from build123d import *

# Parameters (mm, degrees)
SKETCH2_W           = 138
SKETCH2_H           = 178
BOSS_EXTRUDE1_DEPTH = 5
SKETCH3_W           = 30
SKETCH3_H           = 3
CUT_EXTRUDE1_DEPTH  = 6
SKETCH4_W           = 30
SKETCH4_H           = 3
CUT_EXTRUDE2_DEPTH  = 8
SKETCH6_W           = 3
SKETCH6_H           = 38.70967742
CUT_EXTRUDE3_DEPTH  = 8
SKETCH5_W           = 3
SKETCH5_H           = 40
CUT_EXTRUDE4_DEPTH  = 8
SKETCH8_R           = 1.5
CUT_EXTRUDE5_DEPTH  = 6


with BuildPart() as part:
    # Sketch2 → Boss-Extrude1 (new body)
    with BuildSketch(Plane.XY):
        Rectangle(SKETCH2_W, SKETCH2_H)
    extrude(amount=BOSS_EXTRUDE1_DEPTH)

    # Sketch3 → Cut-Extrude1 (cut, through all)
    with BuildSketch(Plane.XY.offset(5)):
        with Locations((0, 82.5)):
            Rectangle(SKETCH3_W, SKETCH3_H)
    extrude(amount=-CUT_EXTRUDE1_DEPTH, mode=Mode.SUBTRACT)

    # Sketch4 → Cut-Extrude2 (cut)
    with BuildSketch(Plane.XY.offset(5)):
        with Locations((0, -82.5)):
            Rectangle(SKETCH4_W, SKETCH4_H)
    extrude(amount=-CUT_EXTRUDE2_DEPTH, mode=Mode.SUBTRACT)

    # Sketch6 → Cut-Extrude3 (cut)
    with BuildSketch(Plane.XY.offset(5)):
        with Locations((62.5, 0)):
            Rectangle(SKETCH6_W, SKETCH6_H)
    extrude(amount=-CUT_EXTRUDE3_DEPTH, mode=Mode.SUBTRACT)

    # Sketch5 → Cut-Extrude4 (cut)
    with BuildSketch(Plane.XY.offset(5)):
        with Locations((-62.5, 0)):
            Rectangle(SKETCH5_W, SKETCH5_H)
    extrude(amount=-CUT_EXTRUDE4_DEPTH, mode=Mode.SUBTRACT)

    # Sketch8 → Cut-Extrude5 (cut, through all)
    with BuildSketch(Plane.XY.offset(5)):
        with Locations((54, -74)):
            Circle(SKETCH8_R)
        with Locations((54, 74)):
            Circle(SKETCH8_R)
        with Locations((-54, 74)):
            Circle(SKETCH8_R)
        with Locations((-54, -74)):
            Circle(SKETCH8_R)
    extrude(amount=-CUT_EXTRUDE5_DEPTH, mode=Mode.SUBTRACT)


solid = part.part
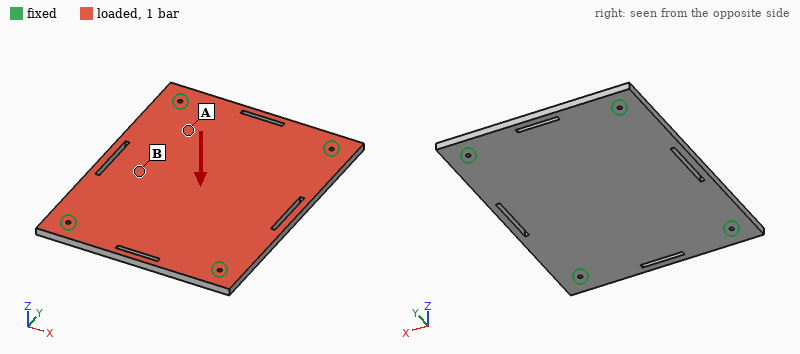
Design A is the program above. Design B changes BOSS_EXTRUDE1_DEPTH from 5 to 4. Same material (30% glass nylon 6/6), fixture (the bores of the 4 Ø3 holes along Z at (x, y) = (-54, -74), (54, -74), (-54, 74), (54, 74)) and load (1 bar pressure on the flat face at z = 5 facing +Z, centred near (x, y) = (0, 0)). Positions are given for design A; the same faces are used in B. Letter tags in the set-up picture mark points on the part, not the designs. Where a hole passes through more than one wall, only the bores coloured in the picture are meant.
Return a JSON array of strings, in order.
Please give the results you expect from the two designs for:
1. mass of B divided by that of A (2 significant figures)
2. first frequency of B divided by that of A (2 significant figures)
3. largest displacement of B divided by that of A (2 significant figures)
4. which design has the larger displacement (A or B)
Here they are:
["0.80", "0.82", "1.9", "B"]
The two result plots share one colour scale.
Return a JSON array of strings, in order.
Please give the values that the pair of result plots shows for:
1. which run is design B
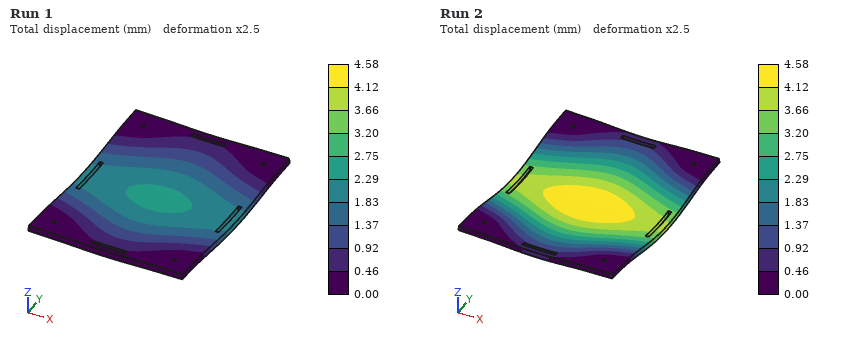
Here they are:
["Run 2"]
